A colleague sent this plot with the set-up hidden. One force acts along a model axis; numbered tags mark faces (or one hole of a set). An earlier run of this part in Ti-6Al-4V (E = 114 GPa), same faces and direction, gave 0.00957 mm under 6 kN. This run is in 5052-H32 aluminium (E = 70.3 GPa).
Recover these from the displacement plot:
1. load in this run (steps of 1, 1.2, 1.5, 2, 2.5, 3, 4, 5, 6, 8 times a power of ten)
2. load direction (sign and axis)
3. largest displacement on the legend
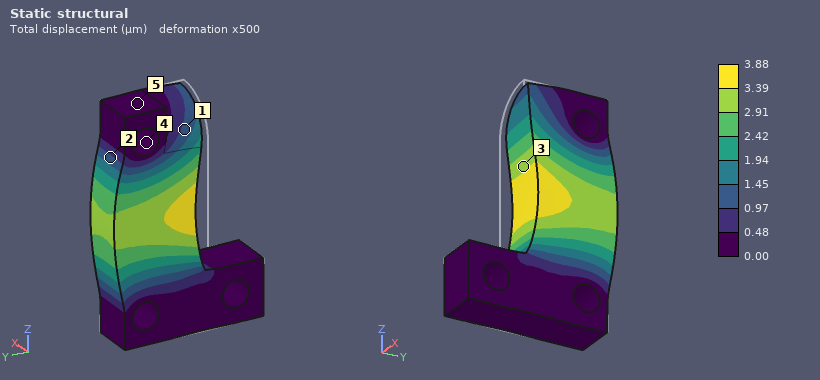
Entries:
1.5 kN
+Y
3.88 µm
